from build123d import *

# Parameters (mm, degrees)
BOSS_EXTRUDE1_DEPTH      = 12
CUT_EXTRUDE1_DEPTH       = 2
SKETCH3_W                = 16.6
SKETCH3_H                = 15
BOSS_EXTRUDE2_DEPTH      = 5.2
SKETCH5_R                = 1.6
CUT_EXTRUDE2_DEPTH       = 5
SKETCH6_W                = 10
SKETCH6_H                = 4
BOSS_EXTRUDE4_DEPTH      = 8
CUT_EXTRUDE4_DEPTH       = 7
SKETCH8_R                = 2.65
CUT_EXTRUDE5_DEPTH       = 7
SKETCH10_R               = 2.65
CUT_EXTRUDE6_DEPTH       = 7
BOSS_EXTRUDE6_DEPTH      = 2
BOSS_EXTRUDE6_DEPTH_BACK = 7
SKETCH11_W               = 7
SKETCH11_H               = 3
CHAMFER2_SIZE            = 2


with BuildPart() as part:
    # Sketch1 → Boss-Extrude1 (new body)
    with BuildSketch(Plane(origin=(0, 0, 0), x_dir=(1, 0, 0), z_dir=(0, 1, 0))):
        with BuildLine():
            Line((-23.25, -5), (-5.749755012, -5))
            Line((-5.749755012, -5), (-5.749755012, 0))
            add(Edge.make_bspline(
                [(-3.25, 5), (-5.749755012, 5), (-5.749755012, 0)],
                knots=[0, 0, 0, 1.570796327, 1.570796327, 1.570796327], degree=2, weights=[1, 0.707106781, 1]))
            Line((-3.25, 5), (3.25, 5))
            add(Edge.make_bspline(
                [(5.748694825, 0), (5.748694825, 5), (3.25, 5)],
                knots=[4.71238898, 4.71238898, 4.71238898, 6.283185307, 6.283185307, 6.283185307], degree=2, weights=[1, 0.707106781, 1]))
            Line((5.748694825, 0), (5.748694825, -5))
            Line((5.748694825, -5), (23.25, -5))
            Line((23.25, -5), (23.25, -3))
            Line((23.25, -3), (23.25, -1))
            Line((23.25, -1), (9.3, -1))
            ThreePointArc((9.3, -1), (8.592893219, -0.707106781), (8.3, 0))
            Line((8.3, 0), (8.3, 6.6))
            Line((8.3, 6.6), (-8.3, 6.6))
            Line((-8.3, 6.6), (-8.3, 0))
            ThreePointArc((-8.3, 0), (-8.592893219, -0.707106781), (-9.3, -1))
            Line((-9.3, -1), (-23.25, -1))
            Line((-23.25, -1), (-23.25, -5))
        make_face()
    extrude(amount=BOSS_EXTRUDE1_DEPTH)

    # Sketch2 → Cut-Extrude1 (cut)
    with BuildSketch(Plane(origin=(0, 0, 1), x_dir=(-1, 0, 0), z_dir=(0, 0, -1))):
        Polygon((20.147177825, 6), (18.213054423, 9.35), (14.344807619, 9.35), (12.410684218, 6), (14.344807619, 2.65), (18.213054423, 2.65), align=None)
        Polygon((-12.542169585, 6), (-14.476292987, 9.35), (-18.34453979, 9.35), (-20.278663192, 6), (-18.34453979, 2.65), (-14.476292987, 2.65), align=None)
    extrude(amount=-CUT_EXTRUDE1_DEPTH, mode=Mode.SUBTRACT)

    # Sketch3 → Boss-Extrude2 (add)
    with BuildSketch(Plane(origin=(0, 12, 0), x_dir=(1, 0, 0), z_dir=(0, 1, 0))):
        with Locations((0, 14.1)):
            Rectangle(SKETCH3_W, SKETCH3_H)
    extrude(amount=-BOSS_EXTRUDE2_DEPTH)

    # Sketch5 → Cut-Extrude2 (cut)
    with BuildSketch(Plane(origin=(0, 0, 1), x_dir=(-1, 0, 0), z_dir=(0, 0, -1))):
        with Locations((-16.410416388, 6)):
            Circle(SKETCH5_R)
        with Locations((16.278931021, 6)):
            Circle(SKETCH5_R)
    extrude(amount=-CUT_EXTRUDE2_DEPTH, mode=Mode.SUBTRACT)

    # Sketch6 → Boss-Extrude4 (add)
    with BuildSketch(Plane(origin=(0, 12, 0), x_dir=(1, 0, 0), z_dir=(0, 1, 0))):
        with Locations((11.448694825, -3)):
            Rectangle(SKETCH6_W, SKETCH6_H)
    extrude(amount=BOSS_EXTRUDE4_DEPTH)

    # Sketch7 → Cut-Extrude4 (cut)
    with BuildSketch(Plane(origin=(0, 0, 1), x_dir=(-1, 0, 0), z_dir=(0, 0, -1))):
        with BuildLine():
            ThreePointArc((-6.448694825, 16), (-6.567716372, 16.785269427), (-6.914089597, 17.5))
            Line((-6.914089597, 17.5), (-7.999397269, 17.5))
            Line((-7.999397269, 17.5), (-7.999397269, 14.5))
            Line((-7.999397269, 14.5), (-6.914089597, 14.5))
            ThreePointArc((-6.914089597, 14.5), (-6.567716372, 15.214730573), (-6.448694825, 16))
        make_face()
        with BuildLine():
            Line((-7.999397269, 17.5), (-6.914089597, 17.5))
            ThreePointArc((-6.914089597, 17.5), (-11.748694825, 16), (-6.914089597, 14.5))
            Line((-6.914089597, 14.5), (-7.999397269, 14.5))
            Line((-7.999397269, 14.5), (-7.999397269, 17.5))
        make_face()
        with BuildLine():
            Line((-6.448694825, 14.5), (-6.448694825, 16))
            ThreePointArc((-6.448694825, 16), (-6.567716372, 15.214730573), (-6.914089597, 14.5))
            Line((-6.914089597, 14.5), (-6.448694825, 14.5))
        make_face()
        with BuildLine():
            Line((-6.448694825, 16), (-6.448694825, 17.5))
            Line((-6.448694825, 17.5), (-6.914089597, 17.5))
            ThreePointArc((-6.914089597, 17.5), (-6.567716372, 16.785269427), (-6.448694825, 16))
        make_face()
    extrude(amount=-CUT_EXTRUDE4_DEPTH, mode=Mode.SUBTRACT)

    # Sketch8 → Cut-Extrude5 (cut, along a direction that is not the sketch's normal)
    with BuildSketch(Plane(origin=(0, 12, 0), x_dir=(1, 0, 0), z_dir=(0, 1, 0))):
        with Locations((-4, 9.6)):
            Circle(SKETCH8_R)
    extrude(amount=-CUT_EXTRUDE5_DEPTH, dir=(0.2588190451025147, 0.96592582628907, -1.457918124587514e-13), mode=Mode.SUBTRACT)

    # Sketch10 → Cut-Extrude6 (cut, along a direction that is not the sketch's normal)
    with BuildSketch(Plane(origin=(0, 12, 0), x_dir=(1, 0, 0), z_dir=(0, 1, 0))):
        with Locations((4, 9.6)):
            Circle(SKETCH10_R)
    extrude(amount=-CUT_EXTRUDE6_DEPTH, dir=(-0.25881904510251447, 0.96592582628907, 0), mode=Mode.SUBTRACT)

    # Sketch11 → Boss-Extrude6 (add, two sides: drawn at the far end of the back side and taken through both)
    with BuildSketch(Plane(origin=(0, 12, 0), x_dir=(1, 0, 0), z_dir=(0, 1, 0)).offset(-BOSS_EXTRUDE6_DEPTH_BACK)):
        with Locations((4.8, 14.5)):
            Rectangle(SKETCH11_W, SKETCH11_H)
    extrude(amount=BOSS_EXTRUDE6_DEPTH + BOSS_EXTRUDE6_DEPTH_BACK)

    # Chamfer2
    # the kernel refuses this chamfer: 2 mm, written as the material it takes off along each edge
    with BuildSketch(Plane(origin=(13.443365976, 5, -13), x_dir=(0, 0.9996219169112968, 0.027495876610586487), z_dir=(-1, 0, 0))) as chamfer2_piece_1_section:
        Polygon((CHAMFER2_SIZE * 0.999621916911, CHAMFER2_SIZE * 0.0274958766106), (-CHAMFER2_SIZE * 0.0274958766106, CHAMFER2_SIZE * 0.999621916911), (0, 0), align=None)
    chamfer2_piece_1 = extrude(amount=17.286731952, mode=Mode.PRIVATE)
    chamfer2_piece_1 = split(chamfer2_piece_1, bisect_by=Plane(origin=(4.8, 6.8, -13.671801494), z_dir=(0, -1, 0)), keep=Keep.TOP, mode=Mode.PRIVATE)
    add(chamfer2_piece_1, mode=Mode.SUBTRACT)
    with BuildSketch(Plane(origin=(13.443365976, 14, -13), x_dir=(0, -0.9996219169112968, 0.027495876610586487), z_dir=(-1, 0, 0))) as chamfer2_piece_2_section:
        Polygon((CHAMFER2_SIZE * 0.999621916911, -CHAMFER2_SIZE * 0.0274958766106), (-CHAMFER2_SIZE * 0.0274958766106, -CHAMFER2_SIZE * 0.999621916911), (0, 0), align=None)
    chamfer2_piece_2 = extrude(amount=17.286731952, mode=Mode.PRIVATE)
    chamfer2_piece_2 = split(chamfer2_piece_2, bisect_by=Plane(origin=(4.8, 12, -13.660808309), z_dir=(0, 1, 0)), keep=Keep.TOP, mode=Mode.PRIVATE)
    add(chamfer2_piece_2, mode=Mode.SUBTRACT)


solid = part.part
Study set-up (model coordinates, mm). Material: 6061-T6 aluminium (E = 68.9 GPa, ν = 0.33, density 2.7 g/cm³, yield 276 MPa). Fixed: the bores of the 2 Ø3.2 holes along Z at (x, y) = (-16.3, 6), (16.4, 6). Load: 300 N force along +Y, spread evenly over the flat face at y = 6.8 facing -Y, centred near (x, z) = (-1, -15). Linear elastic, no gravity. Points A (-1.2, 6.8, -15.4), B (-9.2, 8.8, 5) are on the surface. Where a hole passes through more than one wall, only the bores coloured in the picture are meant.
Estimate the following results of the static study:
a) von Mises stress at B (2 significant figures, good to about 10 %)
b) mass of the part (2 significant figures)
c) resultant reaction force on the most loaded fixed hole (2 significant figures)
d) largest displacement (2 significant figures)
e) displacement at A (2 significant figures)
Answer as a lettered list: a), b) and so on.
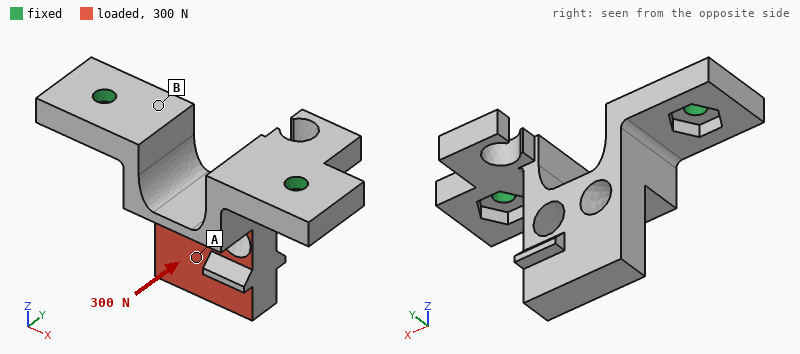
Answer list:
a) 62 MPa
b) 9.7 g
c) 150 N
d) 0.27 mm
e) 0.19 mm
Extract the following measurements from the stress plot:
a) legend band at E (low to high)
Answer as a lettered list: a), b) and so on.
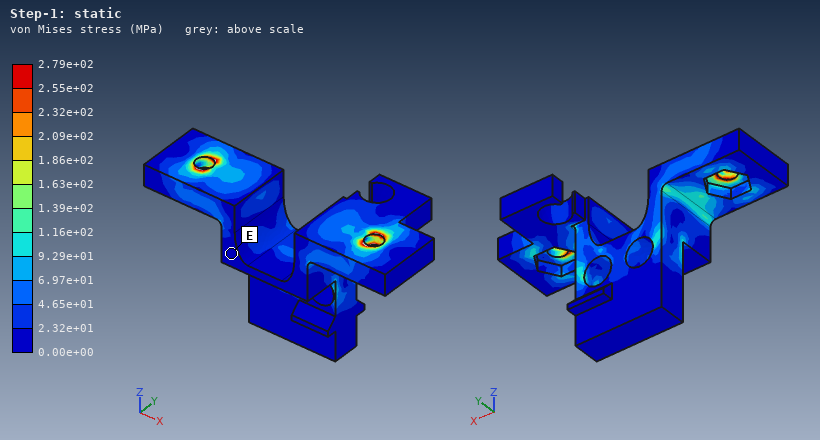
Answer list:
a) 0.00e+00 to 2.32e+01 MPa
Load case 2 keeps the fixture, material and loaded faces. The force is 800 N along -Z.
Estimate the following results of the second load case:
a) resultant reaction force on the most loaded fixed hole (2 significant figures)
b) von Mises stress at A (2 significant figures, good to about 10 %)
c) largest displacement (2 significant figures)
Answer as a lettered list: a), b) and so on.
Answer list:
a) 530 N
b) 29 MPa
c) 45 µm
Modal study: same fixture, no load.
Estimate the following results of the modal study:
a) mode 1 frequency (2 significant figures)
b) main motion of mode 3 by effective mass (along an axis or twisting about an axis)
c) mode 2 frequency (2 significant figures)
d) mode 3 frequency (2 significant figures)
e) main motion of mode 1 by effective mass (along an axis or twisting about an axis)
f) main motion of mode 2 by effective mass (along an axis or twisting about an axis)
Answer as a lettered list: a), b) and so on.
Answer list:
a) 3300 Hz
b) along Z
c) 7800 Hz
d) 11 kHz
e) along Y
f) along X
